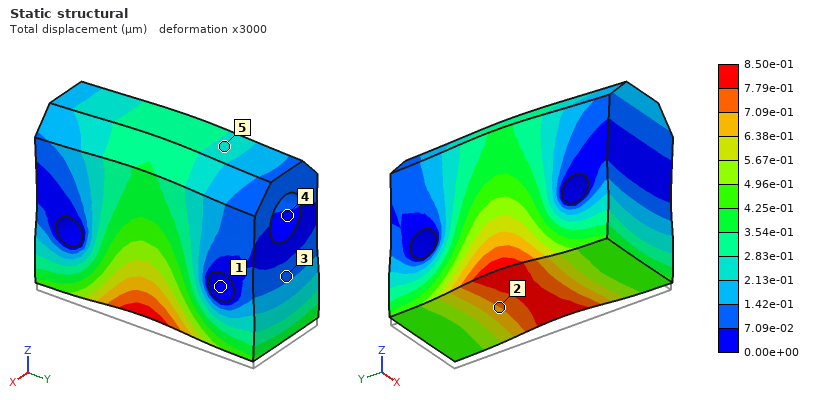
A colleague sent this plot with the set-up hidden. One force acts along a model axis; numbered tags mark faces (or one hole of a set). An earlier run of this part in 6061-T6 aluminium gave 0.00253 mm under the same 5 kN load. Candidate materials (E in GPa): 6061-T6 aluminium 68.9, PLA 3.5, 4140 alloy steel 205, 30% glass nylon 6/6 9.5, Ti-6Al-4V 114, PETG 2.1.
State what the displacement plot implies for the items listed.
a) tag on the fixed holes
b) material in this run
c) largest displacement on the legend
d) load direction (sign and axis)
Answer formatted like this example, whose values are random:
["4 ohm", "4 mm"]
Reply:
["1", "4140 alloy steel", "8.50e-01 µm", "+Z"]
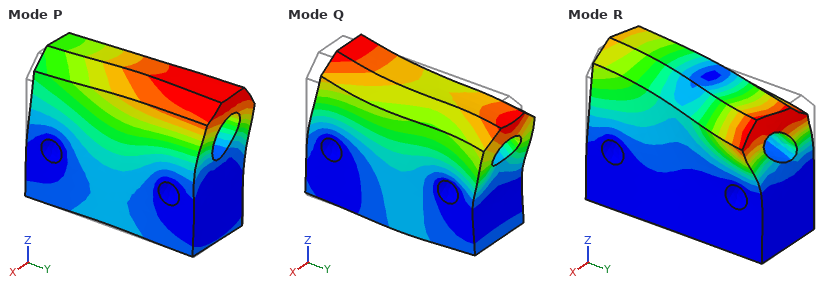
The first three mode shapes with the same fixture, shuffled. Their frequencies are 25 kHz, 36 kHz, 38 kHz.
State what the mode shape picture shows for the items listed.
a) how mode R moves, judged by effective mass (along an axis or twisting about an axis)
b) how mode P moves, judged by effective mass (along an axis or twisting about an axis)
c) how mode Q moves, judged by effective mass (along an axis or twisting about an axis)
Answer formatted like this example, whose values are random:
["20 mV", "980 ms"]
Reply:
["twisting about Z", "along X", "along Y"]
